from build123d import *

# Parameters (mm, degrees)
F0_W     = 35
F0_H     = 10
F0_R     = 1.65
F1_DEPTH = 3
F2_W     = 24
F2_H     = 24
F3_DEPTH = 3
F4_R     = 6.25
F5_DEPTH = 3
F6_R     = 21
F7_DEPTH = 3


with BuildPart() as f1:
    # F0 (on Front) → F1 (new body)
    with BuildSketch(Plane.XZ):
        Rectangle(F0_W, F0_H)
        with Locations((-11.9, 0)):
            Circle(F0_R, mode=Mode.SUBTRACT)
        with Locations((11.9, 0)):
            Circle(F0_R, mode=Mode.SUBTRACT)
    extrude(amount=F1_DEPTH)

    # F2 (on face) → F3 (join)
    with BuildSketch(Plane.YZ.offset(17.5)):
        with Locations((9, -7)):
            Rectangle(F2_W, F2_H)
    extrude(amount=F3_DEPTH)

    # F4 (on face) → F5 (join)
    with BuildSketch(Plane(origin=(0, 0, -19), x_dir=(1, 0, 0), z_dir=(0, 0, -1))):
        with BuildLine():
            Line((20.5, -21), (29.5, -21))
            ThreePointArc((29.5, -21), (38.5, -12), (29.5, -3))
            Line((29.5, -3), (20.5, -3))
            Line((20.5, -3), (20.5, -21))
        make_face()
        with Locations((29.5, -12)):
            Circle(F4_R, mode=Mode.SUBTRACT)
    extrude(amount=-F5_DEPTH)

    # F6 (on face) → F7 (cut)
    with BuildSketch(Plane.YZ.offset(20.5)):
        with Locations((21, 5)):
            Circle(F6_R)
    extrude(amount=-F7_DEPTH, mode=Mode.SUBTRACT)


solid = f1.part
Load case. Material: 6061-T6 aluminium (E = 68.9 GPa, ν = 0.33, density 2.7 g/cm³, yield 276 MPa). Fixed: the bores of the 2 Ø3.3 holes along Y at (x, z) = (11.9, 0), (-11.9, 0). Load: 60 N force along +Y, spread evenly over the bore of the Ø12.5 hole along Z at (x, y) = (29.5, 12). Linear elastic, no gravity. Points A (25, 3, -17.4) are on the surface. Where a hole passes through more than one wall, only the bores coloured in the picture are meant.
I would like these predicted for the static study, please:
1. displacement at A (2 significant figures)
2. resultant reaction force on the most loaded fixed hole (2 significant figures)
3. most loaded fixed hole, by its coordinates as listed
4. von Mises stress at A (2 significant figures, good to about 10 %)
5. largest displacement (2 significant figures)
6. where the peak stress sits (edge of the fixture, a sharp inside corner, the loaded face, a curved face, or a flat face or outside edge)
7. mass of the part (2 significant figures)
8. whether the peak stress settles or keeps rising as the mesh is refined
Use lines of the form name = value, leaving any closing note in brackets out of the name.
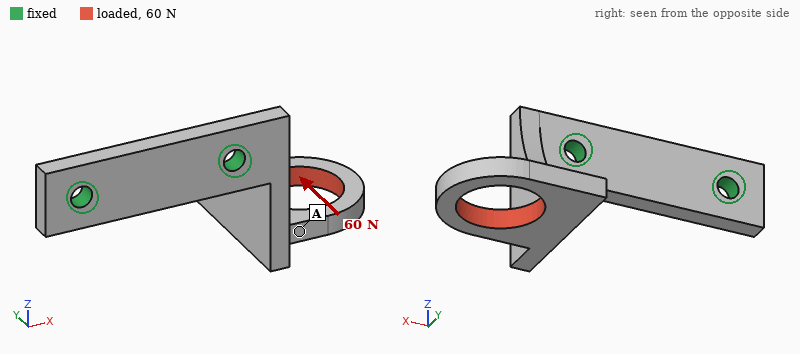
displacement at A = 0.18 mm
resultant reaction force on the most loaded fixed hole = 62 N
most loaded fixed hole, by its coordinates as listed = (11.9, 0)
von Mises stress at A = 14 MPa
largest displacement = 0.40 mm
where the peak stress sits = edge of the fixture
mass of the part = 5.9 g
whether the peak stress settles or keeps rising as the mesh is refined = keeps rising
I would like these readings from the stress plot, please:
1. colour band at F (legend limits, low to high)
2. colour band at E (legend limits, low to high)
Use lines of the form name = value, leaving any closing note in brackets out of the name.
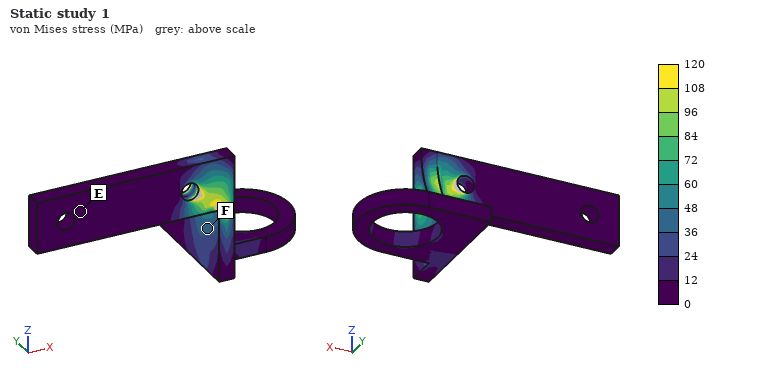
colour band at F = 36 to 48 MPa
colour band at E = 0 to 12 MPa
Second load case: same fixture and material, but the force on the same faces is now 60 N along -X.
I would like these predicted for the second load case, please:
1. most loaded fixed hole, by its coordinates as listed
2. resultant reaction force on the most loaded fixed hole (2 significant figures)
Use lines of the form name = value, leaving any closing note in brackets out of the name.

most loaded fixed hole, by its coordinates as listed = (11.9, 0)
resultant reaction force on the most loaded fixed hole = 60 N
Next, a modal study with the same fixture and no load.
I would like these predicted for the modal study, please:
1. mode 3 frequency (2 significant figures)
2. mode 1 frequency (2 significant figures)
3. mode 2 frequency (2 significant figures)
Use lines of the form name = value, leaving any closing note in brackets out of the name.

mode 3 frequency = 4000 Hz
mode 1 frequency = 1500 Hz
mode 2 frequency = 1900 Hz
